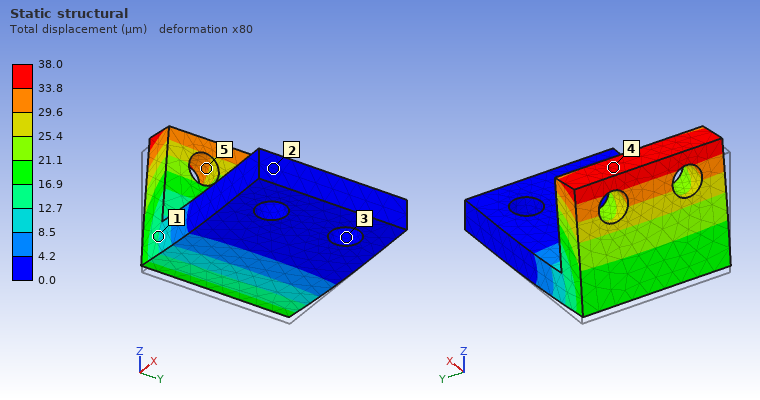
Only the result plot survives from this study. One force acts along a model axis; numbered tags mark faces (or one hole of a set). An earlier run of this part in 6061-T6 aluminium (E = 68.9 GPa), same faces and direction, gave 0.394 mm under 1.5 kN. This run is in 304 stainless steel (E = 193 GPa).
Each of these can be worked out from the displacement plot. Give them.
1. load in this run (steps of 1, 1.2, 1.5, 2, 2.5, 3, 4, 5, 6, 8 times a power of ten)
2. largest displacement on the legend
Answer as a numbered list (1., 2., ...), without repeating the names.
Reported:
1. 400 N
2. 38.0 µm
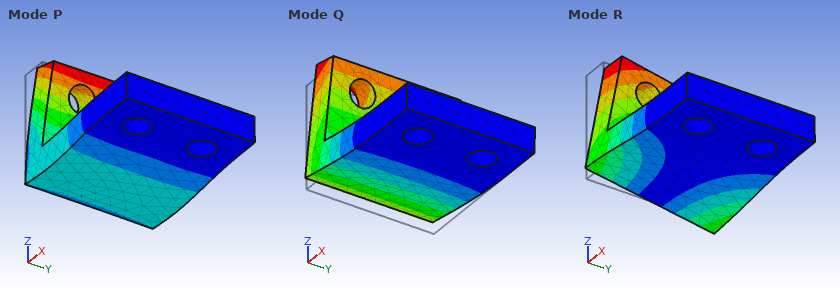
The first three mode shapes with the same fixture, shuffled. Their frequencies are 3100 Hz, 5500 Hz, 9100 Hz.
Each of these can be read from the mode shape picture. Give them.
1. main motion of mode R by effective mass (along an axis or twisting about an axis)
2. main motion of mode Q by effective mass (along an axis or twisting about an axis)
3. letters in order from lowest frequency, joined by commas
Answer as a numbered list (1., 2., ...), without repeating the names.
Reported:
1. along Y
2. along Z
3. Q, R, P
